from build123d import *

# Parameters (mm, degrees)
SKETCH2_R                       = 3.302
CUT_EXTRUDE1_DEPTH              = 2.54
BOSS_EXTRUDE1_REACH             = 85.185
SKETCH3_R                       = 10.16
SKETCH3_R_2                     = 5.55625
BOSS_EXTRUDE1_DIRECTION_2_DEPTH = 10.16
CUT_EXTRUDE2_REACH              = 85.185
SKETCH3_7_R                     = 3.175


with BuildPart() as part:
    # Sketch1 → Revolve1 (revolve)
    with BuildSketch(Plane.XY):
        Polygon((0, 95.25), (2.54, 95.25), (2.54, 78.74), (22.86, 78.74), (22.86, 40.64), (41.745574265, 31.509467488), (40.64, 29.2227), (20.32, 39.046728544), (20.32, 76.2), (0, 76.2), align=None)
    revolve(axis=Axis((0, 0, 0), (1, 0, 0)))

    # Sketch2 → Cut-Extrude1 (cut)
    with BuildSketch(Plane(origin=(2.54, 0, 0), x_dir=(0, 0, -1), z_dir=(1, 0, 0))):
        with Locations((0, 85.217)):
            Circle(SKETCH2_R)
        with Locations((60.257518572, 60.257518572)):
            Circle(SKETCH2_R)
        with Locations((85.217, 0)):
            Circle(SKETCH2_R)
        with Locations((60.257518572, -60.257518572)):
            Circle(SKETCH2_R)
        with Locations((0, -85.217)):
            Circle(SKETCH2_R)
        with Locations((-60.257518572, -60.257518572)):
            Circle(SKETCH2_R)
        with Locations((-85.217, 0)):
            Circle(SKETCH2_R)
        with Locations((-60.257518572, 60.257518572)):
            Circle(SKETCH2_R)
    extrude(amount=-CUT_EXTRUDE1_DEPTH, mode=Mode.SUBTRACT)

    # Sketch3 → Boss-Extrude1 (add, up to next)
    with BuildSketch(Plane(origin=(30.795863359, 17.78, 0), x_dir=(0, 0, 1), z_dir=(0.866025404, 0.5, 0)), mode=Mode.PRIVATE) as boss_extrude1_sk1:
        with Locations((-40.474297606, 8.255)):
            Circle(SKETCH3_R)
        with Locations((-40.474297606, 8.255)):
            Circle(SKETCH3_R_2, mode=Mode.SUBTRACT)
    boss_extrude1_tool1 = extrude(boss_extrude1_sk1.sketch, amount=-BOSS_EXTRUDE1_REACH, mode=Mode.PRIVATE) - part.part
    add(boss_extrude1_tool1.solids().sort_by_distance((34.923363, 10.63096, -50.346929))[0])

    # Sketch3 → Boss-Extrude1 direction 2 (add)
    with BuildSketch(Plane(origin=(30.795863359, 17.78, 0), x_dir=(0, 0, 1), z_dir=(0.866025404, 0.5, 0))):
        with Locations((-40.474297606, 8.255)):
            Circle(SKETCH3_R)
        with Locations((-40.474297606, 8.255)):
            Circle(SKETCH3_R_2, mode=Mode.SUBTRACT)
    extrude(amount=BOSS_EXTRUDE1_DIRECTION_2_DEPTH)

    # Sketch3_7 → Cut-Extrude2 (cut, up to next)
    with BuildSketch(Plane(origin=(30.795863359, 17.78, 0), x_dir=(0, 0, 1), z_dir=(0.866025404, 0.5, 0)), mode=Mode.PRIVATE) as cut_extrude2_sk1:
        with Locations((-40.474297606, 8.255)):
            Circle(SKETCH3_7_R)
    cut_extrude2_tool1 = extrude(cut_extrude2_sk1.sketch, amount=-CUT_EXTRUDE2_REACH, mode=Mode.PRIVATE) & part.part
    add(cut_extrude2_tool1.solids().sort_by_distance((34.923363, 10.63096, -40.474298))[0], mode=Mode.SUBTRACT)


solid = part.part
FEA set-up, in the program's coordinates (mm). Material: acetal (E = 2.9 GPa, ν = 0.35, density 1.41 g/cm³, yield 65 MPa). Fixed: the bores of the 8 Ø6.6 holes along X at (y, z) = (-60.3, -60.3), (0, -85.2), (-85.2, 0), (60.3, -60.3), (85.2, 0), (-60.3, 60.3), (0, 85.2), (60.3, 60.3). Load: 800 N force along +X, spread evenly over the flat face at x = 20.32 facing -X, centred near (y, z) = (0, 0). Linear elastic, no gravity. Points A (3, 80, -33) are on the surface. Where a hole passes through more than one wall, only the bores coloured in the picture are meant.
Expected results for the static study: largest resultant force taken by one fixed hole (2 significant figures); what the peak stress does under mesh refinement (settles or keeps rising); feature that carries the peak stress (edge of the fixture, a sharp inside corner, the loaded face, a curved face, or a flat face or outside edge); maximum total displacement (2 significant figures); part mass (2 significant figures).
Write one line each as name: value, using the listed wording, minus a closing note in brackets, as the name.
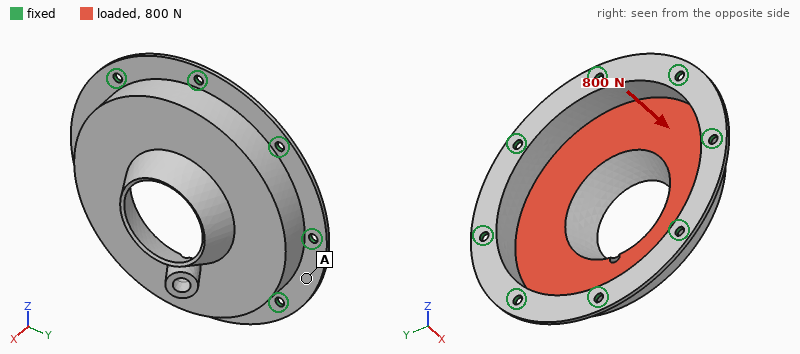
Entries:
largest resultant force taken by one fixed hole: 120 N
what the peak stress does under mesh refinement: keeps rising
feature that carries the peak stress: edge of the fixture
maximum total displacement: 1.5 mm
part mass: 140 g
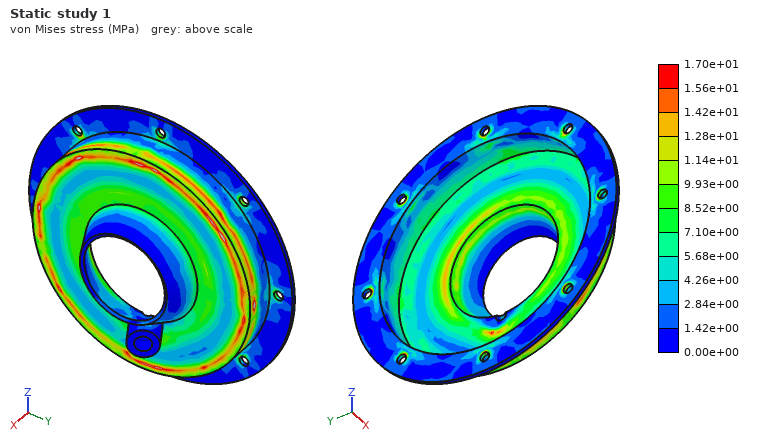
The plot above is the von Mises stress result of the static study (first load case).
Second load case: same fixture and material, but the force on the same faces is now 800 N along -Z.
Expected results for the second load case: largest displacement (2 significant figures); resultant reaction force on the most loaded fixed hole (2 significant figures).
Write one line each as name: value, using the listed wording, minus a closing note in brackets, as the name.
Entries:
largest displacement: 0.10 mm
resultant reaction force on the most loaded fixed hole: 160 N
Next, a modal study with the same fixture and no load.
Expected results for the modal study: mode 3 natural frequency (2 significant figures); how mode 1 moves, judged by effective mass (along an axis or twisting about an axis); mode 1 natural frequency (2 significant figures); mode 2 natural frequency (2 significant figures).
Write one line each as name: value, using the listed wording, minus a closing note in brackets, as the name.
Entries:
mode 3 natural frequency: 630 Hz
how mode 1 moves, judged by effective mass: along X
mode 1 natural frequency: 430 Hz
mode 2 natural frequency: 610 Hz
